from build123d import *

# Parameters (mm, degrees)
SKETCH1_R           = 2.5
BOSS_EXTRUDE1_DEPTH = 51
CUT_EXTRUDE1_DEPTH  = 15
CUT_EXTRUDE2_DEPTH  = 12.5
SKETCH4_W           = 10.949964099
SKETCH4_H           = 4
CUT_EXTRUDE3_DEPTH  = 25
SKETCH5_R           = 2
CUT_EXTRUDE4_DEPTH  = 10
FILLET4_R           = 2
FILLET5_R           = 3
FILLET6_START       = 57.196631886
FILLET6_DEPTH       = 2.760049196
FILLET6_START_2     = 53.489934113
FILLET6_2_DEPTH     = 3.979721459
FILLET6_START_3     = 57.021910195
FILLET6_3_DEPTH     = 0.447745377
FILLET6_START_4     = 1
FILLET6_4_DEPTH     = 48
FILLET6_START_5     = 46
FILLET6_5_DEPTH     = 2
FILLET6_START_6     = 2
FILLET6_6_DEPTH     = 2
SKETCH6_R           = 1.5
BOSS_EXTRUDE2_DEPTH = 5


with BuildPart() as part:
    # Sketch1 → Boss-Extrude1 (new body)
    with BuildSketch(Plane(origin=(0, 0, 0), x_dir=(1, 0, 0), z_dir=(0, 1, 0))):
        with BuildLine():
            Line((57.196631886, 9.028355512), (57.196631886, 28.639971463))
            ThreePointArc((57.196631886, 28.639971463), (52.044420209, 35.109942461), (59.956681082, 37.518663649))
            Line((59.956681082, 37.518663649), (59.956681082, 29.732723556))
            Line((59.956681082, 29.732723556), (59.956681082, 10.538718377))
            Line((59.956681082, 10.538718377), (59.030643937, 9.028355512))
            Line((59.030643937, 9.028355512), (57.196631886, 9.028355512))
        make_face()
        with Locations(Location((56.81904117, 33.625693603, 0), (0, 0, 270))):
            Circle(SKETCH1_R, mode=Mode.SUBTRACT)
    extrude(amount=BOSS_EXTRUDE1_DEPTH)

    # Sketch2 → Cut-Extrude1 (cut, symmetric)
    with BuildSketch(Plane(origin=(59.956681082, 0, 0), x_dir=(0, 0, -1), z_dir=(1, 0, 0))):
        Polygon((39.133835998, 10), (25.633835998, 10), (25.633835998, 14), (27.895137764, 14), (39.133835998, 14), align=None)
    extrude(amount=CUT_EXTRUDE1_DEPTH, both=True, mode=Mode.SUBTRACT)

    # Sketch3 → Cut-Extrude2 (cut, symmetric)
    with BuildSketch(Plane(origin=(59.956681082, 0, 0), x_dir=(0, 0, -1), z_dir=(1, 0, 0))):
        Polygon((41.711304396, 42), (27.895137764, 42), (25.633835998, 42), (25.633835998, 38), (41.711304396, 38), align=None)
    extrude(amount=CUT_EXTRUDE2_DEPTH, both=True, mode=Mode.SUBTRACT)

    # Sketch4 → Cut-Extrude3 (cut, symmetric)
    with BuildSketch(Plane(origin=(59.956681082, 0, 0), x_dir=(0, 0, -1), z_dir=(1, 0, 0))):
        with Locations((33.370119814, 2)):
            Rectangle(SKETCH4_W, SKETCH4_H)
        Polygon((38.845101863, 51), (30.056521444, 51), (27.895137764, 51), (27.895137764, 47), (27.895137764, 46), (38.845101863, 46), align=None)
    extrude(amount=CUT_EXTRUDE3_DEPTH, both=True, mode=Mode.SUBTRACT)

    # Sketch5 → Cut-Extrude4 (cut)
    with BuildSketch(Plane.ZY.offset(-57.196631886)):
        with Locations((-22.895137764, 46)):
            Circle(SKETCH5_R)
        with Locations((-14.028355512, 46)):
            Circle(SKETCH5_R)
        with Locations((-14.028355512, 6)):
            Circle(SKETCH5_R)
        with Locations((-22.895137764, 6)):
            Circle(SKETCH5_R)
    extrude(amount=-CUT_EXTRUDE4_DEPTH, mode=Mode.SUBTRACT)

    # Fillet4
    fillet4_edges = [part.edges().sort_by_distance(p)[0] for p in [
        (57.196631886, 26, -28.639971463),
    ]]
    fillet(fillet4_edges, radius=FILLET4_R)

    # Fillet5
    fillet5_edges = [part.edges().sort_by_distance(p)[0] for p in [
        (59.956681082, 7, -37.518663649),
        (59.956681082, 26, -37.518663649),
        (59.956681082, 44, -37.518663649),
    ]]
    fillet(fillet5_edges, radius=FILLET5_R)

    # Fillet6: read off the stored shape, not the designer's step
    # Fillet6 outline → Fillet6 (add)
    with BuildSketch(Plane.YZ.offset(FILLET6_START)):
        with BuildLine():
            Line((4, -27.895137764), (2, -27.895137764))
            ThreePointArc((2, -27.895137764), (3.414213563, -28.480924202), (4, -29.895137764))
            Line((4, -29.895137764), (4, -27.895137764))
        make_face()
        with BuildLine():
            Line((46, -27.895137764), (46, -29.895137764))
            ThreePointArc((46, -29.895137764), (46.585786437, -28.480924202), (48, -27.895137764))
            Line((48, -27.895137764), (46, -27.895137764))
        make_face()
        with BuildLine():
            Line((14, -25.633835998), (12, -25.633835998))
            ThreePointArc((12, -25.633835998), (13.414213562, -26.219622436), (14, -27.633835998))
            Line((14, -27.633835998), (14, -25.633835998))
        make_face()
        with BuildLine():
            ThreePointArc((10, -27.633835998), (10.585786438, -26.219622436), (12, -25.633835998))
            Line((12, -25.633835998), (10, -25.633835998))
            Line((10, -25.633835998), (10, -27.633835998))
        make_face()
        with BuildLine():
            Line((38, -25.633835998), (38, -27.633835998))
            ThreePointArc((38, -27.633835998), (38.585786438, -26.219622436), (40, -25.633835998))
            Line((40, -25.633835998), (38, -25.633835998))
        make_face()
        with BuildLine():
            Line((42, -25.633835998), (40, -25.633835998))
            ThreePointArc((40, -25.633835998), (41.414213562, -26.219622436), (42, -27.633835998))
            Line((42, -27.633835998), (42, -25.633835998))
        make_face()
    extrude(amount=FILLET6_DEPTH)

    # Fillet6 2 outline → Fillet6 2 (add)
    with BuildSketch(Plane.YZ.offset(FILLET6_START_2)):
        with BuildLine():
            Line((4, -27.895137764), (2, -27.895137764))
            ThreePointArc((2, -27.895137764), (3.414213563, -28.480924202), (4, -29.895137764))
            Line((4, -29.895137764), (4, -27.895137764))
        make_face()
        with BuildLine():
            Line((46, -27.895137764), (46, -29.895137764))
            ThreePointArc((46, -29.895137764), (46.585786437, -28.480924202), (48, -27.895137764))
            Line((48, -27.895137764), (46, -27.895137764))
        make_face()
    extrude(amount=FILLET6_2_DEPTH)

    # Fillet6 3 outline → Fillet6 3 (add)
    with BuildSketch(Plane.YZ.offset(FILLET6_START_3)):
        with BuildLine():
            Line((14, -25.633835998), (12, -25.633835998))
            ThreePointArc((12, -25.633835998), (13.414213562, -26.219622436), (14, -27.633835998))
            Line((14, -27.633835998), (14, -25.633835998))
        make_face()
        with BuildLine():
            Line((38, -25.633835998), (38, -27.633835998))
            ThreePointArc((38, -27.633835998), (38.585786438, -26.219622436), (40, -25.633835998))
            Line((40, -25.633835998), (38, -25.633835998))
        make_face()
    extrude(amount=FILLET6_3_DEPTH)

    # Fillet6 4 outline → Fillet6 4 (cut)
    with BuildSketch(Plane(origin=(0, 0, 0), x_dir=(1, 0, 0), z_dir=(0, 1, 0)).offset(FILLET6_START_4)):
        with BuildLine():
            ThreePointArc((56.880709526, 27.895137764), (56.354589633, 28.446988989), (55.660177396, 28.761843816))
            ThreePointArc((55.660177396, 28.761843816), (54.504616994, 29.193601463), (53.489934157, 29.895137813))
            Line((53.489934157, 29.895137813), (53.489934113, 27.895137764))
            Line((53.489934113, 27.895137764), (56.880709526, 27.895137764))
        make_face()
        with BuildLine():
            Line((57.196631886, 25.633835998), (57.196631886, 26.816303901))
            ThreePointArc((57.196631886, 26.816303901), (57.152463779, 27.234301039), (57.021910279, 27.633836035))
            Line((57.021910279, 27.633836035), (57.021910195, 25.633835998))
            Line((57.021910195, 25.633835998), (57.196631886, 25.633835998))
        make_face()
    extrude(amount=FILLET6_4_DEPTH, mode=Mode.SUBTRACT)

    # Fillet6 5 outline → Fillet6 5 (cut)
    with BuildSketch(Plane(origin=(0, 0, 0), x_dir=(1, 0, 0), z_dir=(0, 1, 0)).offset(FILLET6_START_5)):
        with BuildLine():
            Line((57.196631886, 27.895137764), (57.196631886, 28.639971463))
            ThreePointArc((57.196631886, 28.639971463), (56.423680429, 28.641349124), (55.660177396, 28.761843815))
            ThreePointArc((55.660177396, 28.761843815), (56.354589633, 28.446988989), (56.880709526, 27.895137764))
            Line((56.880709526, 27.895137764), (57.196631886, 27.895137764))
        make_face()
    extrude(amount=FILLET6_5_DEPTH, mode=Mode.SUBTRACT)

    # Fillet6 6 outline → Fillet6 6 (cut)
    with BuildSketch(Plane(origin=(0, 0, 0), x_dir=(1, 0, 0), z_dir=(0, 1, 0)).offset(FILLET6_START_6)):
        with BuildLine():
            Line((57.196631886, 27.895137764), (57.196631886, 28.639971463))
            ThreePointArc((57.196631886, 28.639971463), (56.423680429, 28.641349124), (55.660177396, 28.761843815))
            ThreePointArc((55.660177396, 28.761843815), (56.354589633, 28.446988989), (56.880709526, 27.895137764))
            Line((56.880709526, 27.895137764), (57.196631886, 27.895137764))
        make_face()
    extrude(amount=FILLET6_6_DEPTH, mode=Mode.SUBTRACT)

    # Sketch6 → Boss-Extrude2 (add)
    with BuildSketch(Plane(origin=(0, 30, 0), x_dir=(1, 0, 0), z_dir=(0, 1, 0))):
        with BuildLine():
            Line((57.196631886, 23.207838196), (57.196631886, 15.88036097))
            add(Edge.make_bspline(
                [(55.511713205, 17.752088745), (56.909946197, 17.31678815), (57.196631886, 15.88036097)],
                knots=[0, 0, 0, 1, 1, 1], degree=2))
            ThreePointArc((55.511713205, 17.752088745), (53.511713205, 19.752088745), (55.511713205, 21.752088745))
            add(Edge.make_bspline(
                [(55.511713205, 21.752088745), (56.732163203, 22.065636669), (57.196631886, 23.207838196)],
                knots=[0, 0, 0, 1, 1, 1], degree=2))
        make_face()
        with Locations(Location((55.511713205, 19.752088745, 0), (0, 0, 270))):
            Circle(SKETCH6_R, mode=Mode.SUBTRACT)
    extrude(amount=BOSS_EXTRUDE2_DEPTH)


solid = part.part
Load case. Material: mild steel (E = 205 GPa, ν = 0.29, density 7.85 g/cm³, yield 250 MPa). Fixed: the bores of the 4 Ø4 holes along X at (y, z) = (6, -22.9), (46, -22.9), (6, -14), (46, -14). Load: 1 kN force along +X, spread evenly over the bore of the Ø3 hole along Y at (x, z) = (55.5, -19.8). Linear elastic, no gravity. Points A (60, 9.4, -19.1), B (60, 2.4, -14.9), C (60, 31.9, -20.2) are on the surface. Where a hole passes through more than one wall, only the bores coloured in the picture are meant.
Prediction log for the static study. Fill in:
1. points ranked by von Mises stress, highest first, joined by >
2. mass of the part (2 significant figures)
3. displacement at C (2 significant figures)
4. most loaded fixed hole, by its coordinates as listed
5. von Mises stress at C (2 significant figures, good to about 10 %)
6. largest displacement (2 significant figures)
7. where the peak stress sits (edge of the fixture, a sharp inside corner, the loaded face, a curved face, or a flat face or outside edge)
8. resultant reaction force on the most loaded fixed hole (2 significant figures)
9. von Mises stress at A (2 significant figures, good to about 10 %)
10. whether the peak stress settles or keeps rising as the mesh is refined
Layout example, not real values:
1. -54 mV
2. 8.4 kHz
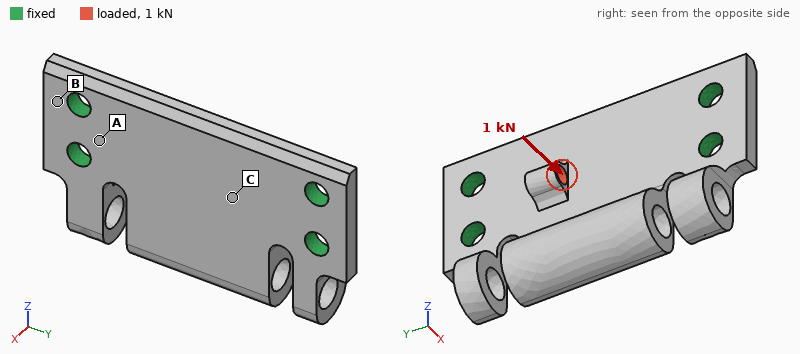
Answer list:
1. C > A > B
2. 33 g
3. 23 µm
4. (46, -22.9)
5. 100 MPa
6. 27 µm
7. edge of the fixture
8. 450 N
9. 57 MPa
10. keeps rising
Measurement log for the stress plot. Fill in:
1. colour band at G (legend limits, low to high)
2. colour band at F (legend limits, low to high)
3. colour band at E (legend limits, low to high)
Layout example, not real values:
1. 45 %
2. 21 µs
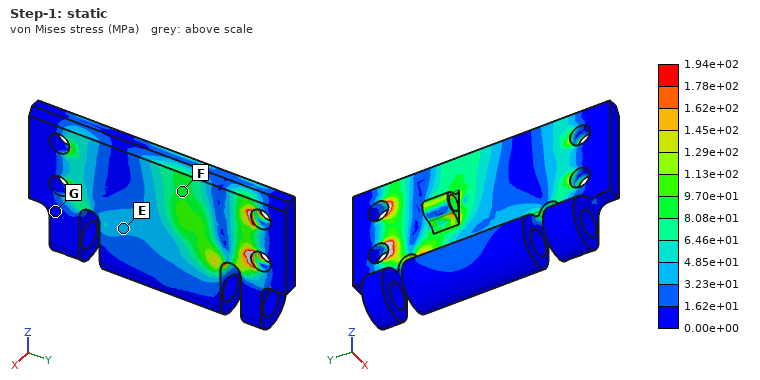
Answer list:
1. 0.00e+00 to 1.62e+01 MPa
2. 8.08e+01 to 9.70e+01 MPa
3. 3.23e+01 to 4.85e+01 MPa
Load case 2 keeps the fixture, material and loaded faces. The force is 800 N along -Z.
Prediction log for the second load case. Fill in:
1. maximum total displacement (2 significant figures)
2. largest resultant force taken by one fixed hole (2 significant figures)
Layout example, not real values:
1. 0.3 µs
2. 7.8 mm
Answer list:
1. 19 µm
2. 430 N
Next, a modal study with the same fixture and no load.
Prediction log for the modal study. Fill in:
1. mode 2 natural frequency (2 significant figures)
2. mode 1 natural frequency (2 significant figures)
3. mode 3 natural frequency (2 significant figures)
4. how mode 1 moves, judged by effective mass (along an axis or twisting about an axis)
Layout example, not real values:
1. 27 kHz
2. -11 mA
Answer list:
1. 8500 Hz
2. 4100 Hz
3. 8800 Hz
4. along X
